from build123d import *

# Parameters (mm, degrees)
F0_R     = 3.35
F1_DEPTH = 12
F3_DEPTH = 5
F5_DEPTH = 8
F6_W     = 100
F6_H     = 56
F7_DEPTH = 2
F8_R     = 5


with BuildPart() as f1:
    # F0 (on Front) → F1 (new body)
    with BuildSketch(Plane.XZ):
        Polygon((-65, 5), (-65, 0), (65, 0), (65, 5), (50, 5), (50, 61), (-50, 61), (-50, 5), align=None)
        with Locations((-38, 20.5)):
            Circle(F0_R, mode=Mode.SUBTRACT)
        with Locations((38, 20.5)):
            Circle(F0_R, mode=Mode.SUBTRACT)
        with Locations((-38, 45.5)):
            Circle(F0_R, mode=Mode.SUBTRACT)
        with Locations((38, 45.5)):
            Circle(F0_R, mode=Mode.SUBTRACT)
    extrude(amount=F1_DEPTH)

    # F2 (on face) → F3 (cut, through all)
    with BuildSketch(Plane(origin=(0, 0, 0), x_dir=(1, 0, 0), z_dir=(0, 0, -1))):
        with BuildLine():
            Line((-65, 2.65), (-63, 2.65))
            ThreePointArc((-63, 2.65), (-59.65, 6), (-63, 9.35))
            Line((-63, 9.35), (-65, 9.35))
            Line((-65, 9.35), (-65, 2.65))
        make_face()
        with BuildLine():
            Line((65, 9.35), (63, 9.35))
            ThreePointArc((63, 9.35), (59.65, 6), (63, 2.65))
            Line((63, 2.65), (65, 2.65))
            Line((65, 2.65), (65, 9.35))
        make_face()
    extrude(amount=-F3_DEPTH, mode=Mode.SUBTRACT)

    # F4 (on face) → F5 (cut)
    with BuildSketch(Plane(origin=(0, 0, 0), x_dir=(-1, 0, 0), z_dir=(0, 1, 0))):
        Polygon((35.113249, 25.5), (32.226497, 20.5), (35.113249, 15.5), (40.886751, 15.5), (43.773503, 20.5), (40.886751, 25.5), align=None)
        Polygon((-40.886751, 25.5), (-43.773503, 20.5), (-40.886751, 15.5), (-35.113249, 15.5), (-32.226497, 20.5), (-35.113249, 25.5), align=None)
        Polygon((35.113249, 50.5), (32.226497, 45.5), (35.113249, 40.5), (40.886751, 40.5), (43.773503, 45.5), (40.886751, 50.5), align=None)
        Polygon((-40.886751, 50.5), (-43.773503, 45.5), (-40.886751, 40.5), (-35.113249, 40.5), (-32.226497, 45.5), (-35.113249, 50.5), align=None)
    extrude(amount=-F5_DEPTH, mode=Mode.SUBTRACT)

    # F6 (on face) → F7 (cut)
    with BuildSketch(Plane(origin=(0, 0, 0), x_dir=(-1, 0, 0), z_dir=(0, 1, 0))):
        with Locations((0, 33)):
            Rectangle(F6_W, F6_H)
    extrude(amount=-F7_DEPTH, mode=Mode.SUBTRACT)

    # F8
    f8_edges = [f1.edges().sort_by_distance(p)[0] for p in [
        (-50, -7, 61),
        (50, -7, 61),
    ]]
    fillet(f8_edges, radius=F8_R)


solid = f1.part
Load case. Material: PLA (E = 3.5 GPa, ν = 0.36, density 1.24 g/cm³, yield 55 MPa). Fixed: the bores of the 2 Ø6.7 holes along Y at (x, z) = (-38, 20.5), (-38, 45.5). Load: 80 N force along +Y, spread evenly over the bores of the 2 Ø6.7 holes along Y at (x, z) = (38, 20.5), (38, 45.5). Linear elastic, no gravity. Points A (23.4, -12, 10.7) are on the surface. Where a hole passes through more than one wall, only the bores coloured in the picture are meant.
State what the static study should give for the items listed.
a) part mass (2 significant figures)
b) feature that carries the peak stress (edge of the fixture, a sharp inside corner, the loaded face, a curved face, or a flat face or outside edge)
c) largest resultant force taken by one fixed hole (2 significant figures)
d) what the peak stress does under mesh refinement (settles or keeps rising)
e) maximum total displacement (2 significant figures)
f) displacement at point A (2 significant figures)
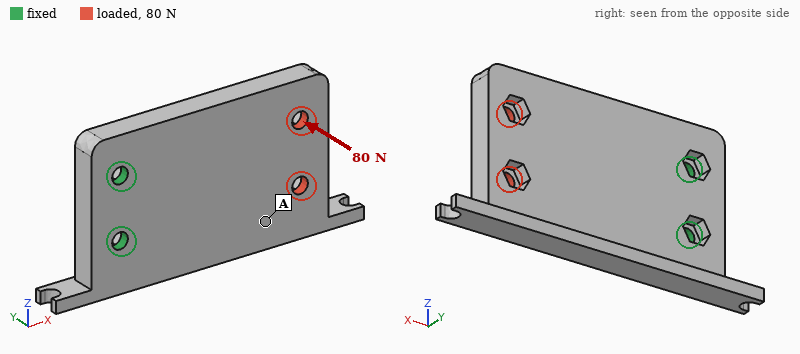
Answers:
75 g
edge of the fixture
69 N
keeps rising
1.7 mm
0.88 mm
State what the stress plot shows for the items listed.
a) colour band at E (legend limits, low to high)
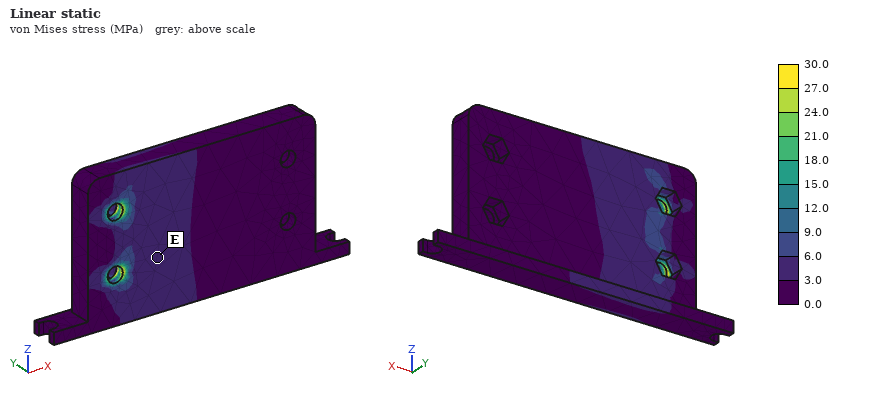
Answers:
3.0 to 6.0 MPa
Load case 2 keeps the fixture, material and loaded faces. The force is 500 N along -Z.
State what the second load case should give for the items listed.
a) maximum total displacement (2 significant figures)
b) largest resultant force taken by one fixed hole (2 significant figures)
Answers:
0.66 mm
1.3 kN
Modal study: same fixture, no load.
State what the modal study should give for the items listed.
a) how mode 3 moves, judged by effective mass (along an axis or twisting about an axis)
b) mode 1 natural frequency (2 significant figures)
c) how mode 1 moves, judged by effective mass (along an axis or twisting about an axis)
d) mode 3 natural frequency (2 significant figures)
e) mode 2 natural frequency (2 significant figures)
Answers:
along Z
250 Hz
along Y
1000 Hz
860 Hz
